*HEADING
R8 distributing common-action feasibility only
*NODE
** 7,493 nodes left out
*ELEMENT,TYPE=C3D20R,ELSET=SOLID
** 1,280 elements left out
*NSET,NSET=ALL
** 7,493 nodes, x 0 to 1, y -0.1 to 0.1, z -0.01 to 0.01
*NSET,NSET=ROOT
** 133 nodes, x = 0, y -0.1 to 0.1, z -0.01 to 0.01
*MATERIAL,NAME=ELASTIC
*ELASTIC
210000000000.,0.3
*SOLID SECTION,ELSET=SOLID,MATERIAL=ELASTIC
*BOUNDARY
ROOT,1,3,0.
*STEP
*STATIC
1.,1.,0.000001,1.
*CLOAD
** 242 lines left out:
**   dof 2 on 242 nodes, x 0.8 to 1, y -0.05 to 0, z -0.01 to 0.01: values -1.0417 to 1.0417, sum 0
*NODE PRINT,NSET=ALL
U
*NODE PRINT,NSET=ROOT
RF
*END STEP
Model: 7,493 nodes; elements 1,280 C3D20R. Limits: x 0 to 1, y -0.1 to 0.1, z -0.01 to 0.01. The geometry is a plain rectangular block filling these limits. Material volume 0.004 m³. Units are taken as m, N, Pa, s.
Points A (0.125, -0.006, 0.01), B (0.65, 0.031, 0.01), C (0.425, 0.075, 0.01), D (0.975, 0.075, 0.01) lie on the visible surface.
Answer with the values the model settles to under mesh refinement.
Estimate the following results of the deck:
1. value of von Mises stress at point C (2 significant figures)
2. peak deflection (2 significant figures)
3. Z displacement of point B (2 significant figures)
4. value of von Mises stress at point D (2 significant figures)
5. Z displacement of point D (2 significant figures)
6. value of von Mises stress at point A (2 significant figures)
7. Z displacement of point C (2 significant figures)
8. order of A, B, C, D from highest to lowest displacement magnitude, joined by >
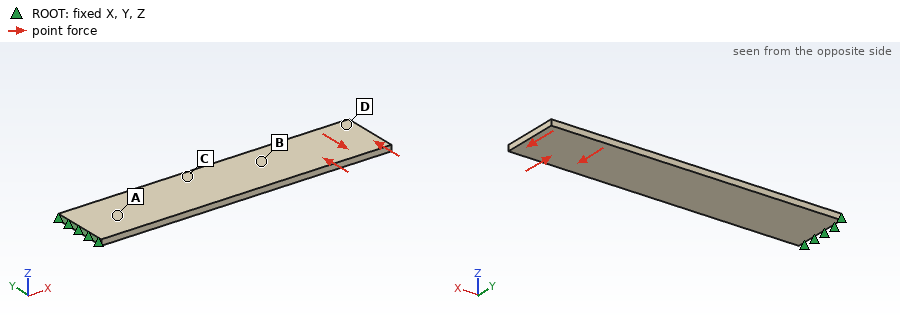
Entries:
68000 Pa
2.1e-06 m
4.7e-07 m
15000 Pa
1.6e-06 m
64000 Pa
7.0e-07 m
D > C > B > A
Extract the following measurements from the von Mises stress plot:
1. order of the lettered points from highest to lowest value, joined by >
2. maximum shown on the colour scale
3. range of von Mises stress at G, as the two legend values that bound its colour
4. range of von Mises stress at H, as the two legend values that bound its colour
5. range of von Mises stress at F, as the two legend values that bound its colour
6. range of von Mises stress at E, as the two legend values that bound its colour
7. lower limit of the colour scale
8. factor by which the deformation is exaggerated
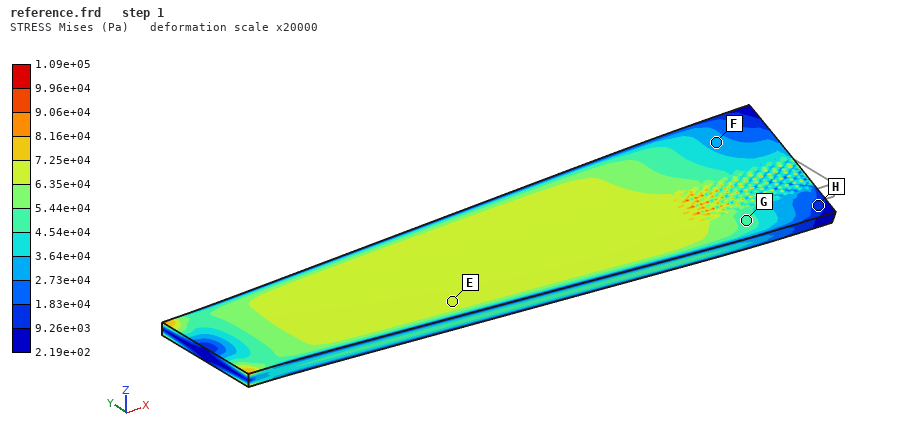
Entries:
E > G > F > H
1.09e+05 Pa
4.54e+04 to 5.44e+04 Pa
9.26e+03 to 1.83e+04 Pa
2.73e+04 to 3.64e+04 Pa
6.35e+04 to 7.25e+04 Pa
2.19e+02 Pa
20000
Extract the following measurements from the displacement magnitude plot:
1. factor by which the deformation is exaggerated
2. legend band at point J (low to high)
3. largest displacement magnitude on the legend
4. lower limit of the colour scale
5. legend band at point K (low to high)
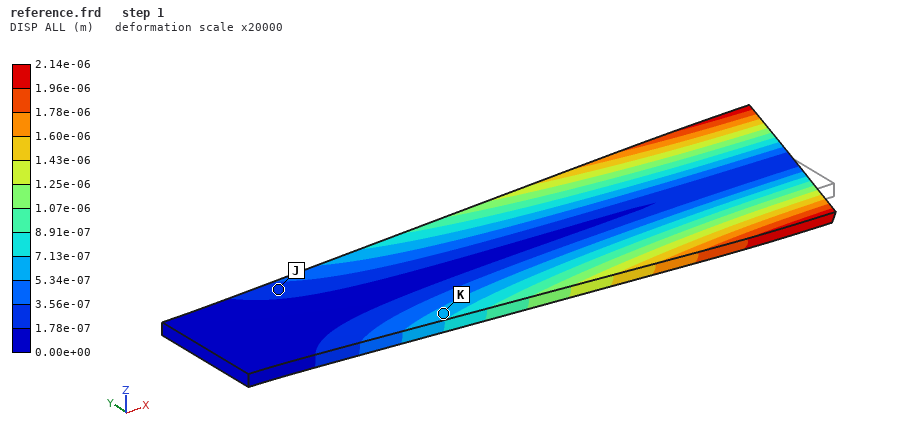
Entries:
20000
1.78e-07 to 3.56e-07 m
2.14e-06 m
0.00e+00 m
5.34e-07 to 7.13e-07 m
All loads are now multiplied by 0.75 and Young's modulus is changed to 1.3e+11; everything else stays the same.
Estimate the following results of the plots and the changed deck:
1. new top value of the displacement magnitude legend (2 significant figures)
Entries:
2.6e-06 m
